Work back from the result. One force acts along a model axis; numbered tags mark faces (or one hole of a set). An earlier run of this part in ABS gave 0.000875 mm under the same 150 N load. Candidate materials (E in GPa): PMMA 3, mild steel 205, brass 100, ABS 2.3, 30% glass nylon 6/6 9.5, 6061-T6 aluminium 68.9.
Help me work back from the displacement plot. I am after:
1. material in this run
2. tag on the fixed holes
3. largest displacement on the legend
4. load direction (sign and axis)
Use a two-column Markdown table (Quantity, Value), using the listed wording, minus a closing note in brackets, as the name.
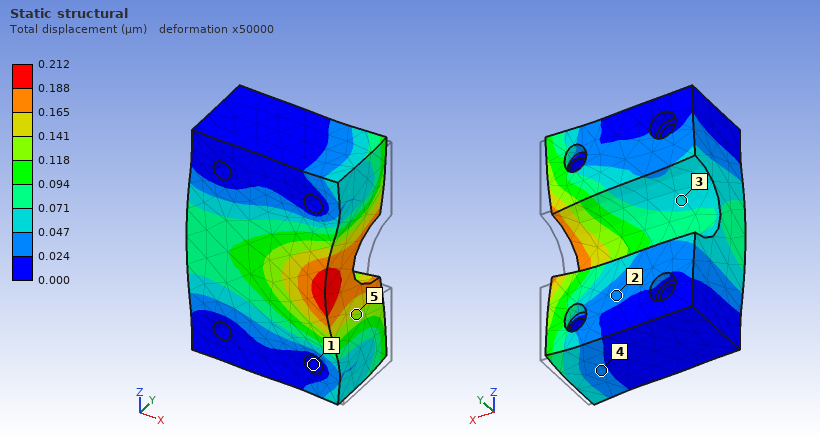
| Quantity | Value |
|---|---|
| material in this run | 30% glass nylon 6/6 |
| tag on the fixed holes | 1 |
| largest displacement on the legend | 0.212 µm |
| load direction | -X |
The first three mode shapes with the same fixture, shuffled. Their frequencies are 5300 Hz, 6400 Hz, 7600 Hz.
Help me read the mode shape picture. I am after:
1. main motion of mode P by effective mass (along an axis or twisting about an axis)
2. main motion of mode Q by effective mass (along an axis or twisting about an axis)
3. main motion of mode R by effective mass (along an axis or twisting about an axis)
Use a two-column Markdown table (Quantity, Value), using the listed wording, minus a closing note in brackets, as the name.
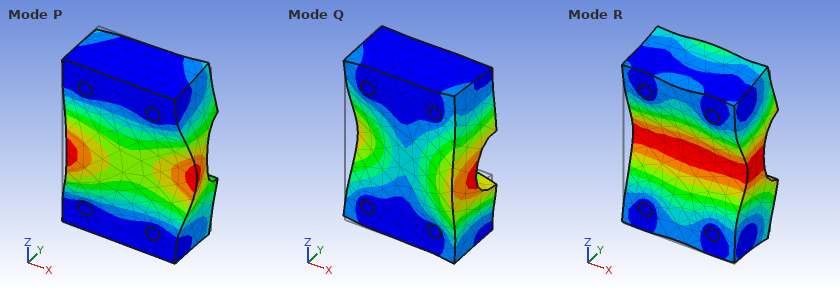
| Quantity | Value |
|---|---|
| main motion of mode P by effective mass | along X |
| main motion of mode Q by effective mass | along X |
| main motion of mode R by effective mass | along Y |
